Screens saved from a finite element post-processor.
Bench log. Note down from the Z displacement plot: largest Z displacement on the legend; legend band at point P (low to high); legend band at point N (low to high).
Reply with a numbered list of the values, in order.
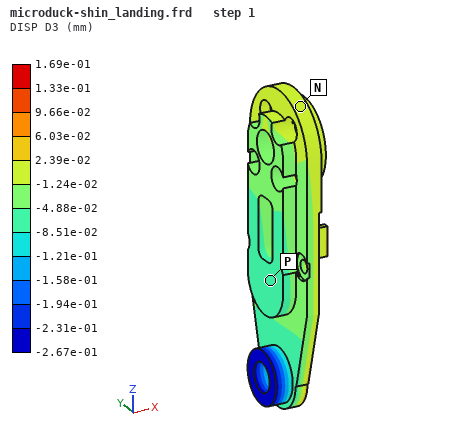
1. 1.69e-01 mm
2. -8.51e-02 to -4.88e-02 mm
3. -1.24e-02 to 2.39e-02 mm
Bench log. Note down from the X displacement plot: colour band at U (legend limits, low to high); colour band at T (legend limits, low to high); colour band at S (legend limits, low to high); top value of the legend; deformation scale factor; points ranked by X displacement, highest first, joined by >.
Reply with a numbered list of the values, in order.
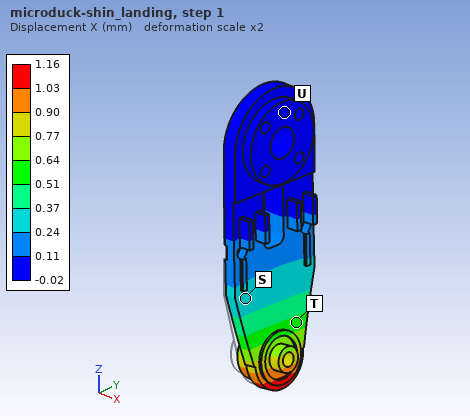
1. -0.02 to 0.11 mm
2. 0.51 to 0.64 mm
3. 0.24 to 0.37 mm
4. 1.16 mm
5. 2
6. T > S > U
